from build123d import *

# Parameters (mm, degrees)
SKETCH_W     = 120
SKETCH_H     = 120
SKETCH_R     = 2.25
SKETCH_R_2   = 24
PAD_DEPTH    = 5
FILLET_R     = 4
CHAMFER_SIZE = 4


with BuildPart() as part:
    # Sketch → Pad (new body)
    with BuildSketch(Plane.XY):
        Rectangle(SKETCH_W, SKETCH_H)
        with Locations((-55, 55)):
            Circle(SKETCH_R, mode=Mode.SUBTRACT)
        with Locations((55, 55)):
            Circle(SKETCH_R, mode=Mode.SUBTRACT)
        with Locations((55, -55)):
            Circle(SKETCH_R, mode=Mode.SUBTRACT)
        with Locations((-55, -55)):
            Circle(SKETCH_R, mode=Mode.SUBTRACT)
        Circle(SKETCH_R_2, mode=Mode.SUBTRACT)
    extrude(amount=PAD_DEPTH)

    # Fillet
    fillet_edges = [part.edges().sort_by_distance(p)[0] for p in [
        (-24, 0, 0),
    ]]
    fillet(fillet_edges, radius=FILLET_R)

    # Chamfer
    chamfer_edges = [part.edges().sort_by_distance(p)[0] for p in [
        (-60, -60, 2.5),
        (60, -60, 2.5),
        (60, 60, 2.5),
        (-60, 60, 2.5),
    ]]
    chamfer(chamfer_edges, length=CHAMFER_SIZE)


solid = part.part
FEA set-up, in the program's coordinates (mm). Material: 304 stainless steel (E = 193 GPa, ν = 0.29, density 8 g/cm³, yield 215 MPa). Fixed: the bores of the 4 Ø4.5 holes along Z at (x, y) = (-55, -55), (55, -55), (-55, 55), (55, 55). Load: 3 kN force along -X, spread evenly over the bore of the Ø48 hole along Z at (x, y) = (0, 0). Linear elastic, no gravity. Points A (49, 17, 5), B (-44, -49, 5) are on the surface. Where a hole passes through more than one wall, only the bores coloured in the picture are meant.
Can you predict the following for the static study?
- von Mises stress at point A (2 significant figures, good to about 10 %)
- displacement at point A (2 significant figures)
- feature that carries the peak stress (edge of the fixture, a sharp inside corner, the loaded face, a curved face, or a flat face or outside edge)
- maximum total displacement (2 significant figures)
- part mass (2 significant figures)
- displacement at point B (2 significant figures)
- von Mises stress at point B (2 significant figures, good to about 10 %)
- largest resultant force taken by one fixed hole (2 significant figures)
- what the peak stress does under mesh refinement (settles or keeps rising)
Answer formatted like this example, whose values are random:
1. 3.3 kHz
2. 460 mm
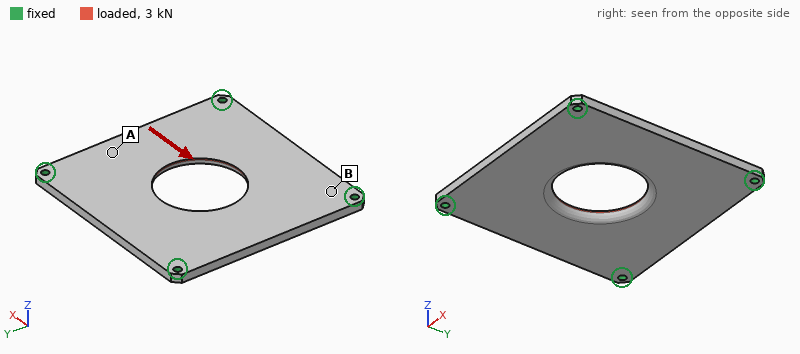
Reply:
1. 3.6 MPa
2. 4.2 µm
3. edge of the fixture
4. 5.4 µm
5. 500 g
6. 0.92 µm
7. 8.8 MPa
8. 850 N
9. keeps rising
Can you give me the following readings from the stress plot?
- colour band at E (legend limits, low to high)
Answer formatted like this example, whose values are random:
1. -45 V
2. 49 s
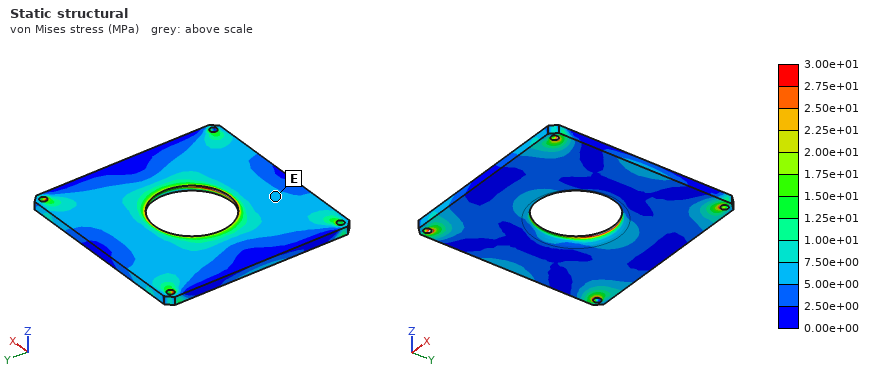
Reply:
1. 5.00e+00 to 7.50e+00 MPa
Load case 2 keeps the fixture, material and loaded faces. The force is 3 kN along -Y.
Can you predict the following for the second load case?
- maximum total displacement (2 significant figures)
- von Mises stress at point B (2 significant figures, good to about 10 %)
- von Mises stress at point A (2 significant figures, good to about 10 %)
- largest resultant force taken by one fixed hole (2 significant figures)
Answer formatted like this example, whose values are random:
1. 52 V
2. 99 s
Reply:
1. 5.4 µm
2. 7.4 MPa
3. 5.1 MPa
4. 850 N
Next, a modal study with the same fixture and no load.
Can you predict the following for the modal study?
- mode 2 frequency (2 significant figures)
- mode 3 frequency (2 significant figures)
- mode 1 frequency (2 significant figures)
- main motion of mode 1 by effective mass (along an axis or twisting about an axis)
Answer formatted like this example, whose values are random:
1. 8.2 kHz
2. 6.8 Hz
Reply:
1. 2100 Hz
2. 2100 Hz
3. 1300 Hz
4. along Z
